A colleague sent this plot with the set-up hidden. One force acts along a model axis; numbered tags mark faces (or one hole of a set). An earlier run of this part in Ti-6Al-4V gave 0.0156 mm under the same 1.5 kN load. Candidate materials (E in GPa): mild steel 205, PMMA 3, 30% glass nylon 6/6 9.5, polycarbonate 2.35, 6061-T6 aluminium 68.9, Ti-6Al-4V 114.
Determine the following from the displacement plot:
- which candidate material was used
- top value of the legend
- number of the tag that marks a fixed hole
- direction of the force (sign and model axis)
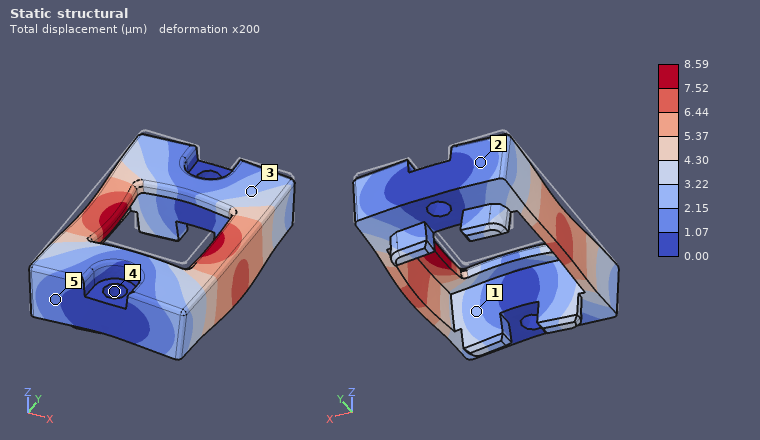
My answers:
mild steel
8.59 µm
4
-Z
